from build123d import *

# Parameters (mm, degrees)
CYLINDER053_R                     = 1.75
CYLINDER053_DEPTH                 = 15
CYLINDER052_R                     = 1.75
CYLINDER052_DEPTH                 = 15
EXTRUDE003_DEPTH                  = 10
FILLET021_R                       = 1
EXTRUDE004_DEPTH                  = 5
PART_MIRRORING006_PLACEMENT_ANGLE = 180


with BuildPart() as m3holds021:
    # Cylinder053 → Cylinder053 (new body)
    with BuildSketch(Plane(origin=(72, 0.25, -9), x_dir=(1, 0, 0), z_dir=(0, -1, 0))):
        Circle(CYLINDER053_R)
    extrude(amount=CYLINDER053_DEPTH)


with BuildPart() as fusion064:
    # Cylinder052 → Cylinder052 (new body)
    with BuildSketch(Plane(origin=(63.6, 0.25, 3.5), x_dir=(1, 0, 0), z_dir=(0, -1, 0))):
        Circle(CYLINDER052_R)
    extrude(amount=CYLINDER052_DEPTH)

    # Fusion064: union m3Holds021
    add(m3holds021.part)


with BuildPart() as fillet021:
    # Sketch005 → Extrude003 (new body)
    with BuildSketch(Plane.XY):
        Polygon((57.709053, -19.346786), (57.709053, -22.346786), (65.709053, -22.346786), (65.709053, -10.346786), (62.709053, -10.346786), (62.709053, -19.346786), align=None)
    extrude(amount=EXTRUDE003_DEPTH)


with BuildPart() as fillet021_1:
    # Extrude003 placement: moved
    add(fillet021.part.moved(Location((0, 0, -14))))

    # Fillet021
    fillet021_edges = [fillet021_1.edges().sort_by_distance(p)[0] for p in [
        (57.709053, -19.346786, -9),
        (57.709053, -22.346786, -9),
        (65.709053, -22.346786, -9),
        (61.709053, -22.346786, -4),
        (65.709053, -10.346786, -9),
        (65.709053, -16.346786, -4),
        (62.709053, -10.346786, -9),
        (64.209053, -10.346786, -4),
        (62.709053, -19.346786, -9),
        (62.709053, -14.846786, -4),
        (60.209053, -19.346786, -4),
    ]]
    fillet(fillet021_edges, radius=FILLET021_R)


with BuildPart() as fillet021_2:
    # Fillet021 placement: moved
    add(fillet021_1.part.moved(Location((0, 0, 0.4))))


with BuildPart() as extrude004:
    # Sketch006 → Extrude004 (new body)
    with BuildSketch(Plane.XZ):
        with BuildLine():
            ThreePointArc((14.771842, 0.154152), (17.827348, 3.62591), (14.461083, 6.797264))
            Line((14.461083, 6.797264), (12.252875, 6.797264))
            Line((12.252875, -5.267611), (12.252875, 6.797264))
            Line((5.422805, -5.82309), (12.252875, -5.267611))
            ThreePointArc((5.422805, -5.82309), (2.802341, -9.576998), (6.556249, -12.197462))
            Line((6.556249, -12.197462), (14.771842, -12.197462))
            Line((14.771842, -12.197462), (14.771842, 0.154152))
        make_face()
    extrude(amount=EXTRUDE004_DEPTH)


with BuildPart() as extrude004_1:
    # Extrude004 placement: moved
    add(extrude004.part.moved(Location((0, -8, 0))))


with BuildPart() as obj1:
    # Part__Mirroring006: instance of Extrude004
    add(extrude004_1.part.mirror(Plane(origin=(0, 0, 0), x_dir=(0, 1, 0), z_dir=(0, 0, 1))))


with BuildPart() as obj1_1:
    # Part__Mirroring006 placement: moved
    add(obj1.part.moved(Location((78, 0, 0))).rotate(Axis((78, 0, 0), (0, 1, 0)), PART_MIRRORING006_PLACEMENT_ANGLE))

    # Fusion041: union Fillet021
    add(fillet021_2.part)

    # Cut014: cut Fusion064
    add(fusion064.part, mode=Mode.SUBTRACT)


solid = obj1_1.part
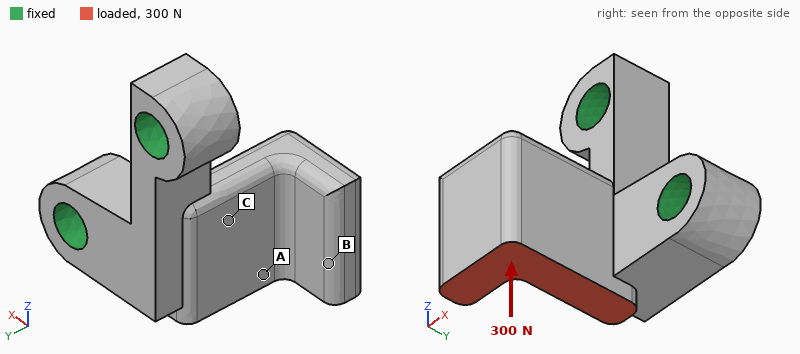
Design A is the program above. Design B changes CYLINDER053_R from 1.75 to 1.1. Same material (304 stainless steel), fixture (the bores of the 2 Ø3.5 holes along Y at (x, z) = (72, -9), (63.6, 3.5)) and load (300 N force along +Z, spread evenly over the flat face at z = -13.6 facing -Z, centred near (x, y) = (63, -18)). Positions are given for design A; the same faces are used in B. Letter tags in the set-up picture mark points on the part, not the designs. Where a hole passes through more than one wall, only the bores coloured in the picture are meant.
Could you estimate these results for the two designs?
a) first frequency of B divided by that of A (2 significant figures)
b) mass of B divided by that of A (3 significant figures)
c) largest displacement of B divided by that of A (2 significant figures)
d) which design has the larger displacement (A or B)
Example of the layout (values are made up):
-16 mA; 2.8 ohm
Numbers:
0.97; 1.03; 1.1; B
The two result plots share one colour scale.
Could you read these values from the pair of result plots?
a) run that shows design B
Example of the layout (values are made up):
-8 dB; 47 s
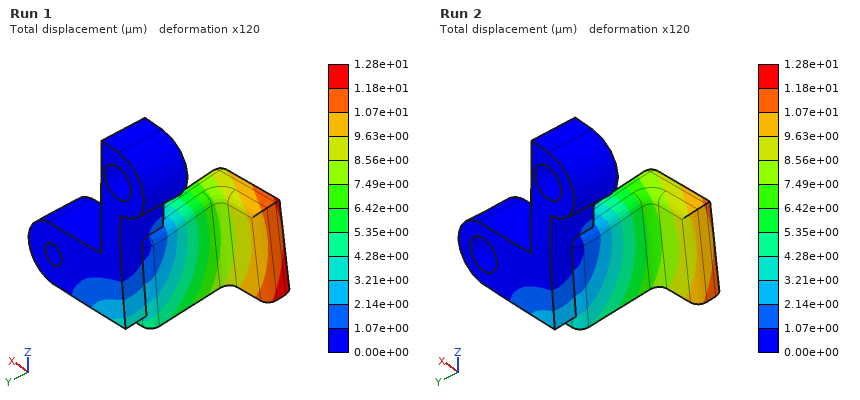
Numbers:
Run 1
